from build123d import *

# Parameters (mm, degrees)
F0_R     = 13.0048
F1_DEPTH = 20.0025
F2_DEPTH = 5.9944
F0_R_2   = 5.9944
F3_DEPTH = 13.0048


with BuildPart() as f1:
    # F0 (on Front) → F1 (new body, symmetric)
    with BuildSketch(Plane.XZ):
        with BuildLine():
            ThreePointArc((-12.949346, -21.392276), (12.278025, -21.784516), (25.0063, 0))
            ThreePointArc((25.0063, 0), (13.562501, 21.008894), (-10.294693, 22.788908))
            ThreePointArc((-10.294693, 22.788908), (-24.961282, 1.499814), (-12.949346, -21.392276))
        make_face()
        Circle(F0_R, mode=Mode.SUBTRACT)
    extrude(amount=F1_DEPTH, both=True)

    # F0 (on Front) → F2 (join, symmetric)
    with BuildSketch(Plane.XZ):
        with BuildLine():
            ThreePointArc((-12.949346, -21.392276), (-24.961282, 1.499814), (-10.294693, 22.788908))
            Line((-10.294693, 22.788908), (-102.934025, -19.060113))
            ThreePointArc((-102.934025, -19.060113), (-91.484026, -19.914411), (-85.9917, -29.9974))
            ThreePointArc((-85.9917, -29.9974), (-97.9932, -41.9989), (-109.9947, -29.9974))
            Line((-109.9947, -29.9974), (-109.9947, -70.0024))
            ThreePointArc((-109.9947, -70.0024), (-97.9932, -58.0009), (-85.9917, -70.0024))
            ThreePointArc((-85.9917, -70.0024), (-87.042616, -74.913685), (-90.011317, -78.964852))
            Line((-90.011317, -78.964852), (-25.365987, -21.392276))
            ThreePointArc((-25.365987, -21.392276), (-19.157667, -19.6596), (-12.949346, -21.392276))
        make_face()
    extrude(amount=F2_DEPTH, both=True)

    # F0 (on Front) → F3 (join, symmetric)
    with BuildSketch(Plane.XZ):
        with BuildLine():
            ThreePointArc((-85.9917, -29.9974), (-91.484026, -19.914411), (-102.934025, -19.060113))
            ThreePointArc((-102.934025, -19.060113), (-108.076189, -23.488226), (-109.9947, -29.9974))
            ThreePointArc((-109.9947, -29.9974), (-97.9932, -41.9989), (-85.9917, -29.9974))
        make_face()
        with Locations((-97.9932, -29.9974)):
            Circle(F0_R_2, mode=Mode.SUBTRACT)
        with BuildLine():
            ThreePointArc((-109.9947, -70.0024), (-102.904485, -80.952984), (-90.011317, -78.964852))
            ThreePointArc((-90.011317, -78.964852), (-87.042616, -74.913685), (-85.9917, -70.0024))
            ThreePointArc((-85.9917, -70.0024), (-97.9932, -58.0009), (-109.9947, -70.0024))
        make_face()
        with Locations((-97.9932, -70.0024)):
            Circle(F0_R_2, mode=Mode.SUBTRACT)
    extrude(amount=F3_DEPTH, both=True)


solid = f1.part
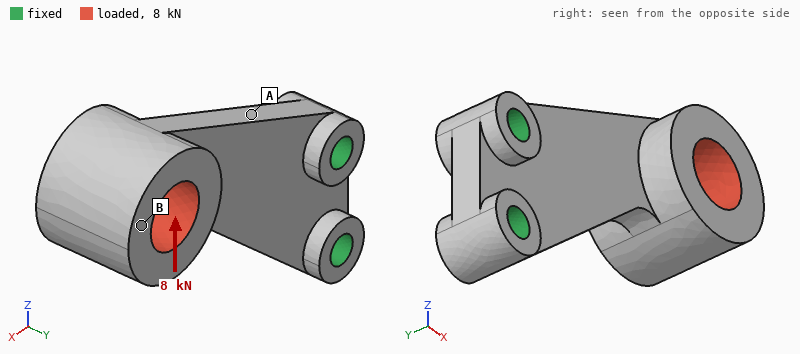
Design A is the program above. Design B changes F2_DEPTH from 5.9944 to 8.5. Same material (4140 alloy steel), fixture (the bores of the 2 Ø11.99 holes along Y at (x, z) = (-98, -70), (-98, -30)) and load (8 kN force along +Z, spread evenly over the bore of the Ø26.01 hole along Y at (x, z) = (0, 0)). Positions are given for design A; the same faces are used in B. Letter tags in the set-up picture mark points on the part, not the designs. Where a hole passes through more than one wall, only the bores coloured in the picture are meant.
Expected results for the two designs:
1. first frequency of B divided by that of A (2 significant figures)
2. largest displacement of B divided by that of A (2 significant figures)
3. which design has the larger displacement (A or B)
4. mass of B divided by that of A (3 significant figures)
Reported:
1.6
0.72
A
1.16
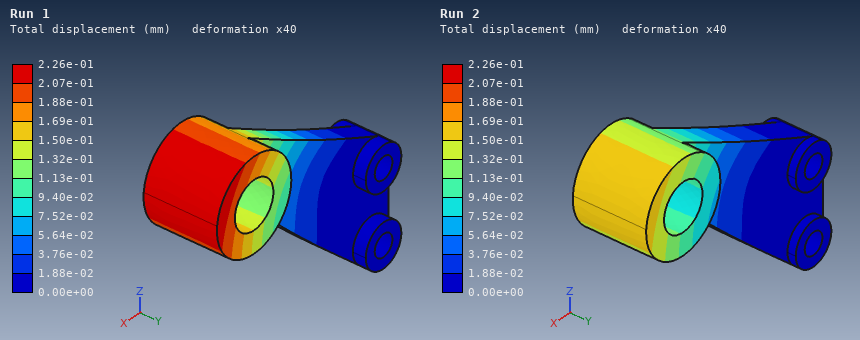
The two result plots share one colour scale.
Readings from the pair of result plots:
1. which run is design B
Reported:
Run 2
